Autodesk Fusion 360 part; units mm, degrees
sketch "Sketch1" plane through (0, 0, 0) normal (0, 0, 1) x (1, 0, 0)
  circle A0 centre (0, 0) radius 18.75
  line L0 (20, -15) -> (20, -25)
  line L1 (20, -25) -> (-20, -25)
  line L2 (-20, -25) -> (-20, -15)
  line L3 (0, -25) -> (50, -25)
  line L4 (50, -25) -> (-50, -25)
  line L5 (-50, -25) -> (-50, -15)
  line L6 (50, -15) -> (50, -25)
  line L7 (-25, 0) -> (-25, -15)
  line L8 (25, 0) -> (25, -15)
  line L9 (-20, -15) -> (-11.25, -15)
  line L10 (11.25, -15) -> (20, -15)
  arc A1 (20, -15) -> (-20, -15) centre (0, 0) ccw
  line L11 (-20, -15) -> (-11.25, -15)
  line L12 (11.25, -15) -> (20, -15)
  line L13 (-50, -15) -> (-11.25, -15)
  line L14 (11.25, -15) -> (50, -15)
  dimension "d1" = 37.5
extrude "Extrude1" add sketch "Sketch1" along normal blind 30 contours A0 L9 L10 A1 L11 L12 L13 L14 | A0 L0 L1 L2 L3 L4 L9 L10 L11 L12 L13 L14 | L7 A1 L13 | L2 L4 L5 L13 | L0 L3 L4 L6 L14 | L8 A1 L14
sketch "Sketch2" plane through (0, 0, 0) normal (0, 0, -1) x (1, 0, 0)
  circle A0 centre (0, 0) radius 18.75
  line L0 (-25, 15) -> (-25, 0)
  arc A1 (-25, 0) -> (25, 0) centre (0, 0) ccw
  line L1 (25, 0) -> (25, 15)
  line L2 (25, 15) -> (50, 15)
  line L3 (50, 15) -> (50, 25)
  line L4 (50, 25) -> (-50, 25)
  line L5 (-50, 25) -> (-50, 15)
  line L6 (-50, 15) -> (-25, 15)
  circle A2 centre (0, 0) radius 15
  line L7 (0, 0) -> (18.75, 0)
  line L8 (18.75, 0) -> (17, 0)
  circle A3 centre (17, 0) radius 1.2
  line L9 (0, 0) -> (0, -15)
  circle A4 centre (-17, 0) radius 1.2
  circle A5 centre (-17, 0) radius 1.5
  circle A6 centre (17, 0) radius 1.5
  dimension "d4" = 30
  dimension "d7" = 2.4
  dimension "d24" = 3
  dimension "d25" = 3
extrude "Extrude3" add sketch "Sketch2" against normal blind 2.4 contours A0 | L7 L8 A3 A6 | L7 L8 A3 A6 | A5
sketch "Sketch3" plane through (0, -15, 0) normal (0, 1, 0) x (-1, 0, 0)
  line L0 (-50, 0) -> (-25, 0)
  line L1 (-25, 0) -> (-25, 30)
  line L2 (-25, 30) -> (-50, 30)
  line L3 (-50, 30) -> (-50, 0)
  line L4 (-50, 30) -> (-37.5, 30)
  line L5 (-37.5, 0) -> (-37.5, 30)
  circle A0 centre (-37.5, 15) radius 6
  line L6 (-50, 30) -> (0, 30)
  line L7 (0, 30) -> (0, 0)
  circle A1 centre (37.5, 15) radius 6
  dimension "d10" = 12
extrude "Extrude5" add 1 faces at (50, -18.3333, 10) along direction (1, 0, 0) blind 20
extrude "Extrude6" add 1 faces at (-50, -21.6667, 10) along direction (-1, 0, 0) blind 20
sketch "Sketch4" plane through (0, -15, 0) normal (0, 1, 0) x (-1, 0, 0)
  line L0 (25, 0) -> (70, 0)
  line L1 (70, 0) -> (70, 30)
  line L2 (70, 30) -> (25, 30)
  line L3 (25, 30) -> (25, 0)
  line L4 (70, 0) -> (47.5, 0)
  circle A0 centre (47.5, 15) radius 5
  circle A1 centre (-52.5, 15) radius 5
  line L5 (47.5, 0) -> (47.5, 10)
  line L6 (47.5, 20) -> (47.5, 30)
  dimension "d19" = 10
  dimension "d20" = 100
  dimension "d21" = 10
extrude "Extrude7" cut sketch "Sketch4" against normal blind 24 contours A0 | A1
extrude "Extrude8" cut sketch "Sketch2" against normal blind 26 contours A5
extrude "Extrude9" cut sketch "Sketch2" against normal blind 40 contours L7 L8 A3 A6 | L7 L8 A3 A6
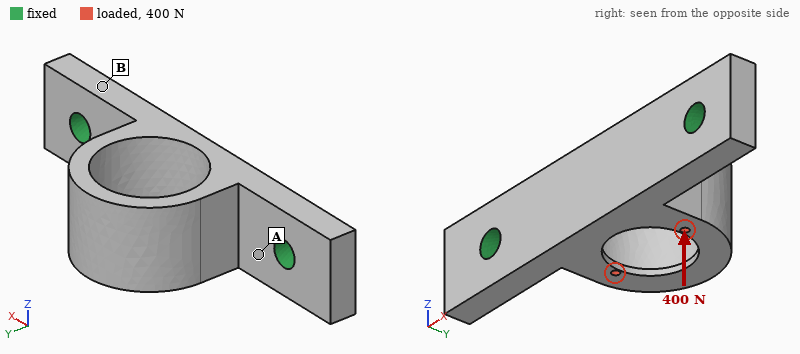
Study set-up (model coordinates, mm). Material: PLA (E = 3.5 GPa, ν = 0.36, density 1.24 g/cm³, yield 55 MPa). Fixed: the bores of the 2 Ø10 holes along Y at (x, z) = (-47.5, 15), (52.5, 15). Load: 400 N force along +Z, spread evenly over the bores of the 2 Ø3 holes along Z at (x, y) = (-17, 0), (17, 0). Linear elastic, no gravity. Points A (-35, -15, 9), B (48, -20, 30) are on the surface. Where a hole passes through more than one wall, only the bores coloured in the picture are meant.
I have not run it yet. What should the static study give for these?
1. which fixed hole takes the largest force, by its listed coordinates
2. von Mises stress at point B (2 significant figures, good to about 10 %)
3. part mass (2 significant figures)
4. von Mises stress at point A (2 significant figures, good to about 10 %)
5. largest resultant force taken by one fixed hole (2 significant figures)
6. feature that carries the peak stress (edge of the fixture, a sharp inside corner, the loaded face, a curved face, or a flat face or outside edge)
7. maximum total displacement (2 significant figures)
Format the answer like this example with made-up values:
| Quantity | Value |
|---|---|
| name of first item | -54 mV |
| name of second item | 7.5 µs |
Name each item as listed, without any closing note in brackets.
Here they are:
| Quantity | Value |
|---|---|
| which fixed hole takes the largest force, by its listed coordinates | (-47.5, 15) |
| von Mises stress at point B | 3.9 MPa |
| part mass | 75 g |
| von Mises stress at point A | 7.9 MPa |
| largest resultant force taken by one fixed hole | 210 N |
| feature that carries the peak stress | the loaded face |
| maximum total displacement | 0.45 mm |
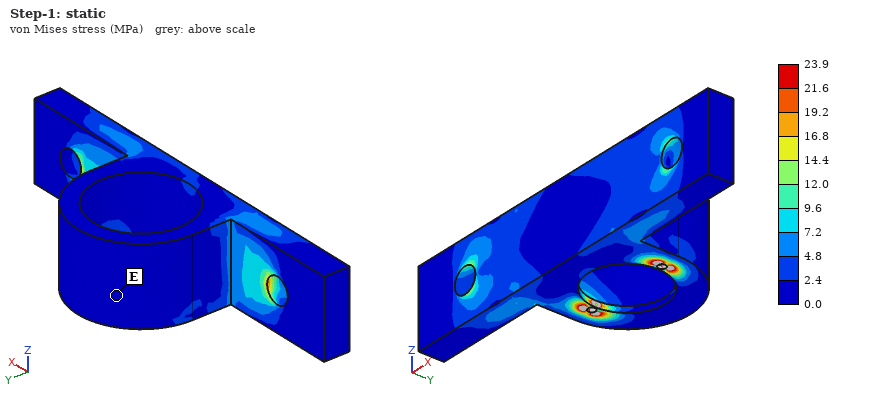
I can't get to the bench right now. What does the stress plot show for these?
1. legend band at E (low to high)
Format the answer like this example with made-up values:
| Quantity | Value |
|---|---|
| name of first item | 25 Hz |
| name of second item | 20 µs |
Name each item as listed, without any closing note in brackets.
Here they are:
| Quantity | Value |
|---|---|
| legend band at E | 0.0 to 2.4 MPa |
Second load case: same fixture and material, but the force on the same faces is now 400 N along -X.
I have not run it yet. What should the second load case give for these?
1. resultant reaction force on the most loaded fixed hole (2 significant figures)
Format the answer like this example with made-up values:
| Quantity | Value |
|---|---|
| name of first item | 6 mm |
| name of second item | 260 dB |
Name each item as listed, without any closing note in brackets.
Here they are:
| Quantity | Value |
|---|---|
| resultant reaction force on the most loaded fixed hole | 240 N |
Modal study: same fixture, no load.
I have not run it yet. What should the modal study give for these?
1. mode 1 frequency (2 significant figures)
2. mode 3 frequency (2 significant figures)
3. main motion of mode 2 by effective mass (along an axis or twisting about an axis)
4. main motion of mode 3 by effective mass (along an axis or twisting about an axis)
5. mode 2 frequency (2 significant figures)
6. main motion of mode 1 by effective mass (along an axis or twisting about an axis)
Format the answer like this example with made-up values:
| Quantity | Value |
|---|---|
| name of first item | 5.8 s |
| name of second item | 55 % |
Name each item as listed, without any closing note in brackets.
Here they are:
| Quantity | Value |
|---|---|
| mode 1 frequency | 930 Hz |
| mode 3 frequency | 1800 Hz |
| main motion of mode 2 by effective mass | along Y |
| main motion of mode 3 by effective mass | along X |
| mode 2 frequency | 1500 Hz |
| main motion of mode 1 by effective mass | along Z |
